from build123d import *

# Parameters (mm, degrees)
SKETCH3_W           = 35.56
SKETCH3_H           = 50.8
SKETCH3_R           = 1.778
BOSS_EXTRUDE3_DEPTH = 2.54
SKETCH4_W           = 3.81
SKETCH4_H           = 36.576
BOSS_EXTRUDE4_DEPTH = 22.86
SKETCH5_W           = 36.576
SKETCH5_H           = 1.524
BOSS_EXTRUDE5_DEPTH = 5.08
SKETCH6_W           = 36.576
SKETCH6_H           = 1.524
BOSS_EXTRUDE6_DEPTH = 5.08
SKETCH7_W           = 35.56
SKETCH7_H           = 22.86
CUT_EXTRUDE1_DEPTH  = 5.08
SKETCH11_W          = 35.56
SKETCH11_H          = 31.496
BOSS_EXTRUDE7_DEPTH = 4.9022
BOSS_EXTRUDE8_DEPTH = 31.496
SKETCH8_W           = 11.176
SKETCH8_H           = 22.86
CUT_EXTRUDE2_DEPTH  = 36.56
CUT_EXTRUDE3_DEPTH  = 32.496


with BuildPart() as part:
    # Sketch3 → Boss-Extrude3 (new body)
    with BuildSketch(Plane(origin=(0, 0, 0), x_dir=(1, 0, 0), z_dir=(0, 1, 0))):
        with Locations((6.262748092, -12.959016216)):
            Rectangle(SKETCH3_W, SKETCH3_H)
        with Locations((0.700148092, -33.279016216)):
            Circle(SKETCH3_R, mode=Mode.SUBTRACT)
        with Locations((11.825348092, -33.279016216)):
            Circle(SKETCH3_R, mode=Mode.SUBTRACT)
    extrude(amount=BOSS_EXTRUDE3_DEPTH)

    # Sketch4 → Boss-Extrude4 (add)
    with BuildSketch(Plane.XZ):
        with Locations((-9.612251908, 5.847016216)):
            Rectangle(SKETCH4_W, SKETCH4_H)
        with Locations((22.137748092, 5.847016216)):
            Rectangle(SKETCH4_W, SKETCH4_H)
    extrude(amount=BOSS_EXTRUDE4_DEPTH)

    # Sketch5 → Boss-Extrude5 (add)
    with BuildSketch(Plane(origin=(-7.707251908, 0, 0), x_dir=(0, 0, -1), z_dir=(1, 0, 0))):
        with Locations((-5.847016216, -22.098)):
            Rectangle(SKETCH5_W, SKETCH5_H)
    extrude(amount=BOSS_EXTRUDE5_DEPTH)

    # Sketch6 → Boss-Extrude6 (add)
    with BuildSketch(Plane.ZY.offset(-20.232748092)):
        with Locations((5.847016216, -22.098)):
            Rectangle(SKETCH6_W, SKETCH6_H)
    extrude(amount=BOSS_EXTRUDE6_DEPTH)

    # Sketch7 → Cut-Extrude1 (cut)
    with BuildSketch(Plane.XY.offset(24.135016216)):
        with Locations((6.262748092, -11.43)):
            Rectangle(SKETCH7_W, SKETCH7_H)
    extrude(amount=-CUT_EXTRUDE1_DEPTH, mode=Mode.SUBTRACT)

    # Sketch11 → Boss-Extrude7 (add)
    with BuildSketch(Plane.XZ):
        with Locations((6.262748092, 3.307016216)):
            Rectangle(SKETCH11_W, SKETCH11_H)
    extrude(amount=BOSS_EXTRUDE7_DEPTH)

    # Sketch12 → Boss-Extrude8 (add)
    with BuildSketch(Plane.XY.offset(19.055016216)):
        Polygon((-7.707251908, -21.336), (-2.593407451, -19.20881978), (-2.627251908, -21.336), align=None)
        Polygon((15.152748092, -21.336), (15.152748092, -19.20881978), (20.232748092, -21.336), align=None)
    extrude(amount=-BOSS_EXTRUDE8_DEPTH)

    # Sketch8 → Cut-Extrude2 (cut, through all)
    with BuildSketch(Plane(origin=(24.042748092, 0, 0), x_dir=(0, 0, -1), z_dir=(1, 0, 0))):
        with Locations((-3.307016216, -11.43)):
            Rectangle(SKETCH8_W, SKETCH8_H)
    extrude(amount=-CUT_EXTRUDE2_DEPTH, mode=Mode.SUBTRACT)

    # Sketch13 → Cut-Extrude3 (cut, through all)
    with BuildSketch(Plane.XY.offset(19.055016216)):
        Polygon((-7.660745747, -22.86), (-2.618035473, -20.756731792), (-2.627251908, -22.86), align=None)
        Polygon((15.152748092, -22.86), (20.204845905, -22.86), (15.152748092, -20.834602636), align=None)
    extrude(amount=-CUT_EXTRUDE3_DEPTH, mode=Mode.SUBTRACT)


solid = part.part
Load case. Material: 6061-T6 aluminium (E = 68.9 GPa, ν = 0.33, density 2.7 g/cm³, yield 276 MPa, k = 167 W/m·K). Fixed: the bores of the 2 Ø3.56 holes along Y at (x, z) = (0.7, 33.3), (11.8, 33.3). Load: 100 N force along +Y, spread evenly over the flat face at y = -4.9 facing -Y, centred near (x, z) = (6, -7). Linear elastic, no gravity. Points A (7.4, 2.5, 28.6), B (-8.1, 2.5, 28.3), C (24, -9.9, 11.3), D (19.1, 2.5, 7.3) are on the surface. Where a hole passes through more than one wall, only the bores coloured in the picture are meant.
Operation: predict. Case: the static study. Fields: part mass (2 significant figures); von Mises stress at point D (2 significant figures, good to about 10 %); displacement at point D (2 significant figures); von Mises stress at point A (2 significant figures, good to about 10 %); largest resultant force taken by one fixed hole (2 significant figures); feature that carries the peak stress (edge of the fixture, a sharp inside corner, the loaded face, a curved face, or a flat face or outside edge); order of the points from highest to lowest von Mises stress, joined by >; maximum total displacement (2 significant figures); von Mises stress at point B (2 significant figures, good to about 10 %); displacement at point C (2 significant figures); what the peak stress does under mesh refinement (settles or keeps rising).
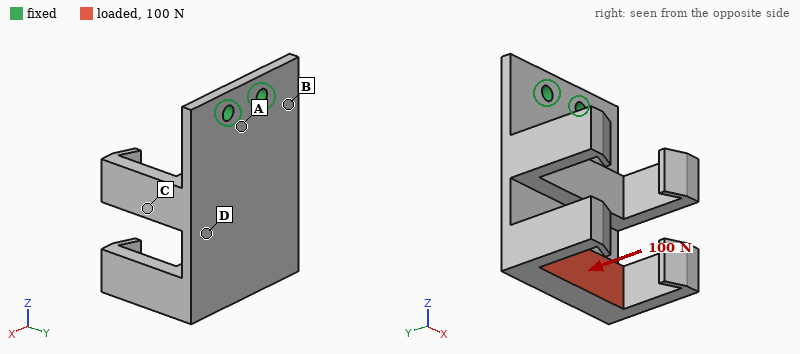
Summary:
30 g
33 MPa
0.28 mm
97 MPa
50 N
edge of the fixture
A > B > D > C
0.78 mm
70 MPa
0.27 mm
keeps rising
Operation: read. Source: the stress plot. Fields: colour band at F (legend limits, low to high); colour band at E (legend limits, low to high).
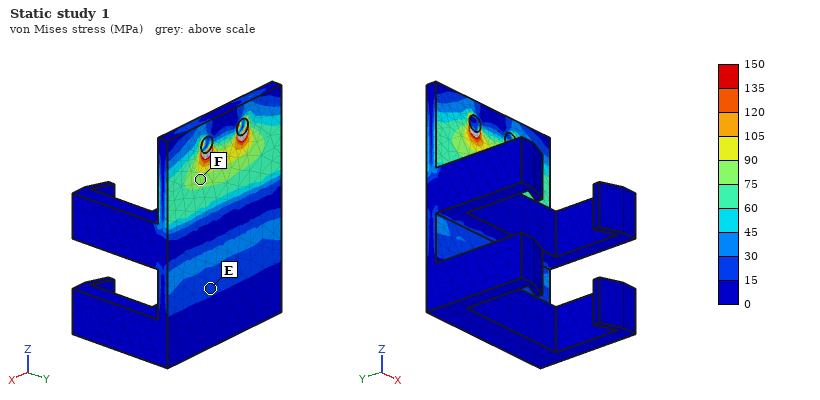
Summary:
75 to 90 MPa
15 to 30 MPa
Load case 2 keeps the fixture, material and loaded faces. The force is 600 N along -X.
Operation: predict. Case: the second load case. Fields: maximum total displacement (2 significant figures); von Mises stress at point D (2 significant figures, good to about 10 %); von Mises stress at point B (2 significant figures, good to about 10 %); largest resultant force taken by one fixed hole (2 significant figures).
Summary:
0.30 mm
39 MPa
39 MPa
1.7 kN
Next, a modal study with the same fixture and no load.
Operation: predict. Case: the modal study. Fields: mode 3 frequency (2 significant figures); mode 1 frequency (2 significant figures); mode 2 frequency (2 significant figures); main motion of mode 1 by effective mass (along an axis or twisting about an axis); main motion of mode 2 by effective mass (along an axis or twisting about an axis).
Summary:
2500 Hz
530 Hz
1500 Hz
along Y
along X
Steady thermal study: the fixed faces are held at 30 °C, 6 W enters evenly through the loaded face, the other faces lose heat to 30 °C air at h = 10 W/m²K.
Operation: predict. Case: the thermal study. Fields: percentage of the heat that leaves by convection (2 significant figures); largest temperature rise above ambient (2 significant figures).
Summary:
9.7 %
14 K
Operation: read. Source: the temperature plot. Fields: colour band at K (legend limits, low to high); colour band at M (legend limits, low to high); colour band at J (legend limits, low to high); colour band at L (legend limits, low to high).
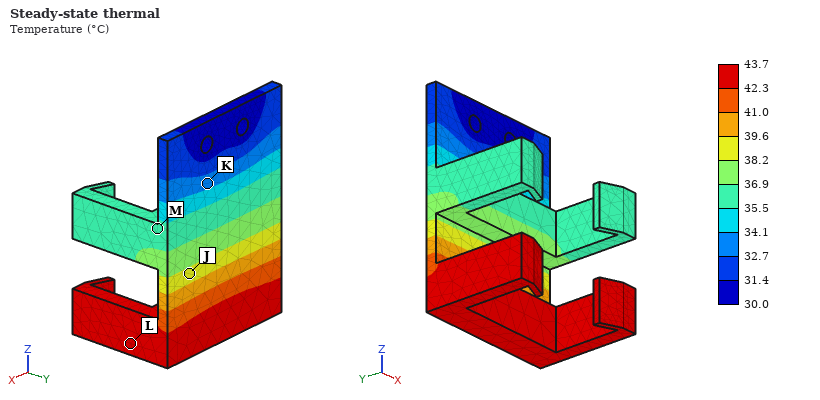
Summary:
32.7 to 34.1 °C
35.5 to 36.9 °C
38.2 to 39.6 °C
42.3 to 43.7 °C
